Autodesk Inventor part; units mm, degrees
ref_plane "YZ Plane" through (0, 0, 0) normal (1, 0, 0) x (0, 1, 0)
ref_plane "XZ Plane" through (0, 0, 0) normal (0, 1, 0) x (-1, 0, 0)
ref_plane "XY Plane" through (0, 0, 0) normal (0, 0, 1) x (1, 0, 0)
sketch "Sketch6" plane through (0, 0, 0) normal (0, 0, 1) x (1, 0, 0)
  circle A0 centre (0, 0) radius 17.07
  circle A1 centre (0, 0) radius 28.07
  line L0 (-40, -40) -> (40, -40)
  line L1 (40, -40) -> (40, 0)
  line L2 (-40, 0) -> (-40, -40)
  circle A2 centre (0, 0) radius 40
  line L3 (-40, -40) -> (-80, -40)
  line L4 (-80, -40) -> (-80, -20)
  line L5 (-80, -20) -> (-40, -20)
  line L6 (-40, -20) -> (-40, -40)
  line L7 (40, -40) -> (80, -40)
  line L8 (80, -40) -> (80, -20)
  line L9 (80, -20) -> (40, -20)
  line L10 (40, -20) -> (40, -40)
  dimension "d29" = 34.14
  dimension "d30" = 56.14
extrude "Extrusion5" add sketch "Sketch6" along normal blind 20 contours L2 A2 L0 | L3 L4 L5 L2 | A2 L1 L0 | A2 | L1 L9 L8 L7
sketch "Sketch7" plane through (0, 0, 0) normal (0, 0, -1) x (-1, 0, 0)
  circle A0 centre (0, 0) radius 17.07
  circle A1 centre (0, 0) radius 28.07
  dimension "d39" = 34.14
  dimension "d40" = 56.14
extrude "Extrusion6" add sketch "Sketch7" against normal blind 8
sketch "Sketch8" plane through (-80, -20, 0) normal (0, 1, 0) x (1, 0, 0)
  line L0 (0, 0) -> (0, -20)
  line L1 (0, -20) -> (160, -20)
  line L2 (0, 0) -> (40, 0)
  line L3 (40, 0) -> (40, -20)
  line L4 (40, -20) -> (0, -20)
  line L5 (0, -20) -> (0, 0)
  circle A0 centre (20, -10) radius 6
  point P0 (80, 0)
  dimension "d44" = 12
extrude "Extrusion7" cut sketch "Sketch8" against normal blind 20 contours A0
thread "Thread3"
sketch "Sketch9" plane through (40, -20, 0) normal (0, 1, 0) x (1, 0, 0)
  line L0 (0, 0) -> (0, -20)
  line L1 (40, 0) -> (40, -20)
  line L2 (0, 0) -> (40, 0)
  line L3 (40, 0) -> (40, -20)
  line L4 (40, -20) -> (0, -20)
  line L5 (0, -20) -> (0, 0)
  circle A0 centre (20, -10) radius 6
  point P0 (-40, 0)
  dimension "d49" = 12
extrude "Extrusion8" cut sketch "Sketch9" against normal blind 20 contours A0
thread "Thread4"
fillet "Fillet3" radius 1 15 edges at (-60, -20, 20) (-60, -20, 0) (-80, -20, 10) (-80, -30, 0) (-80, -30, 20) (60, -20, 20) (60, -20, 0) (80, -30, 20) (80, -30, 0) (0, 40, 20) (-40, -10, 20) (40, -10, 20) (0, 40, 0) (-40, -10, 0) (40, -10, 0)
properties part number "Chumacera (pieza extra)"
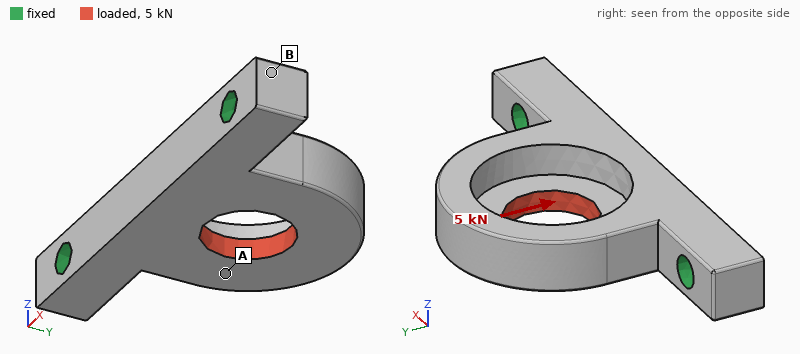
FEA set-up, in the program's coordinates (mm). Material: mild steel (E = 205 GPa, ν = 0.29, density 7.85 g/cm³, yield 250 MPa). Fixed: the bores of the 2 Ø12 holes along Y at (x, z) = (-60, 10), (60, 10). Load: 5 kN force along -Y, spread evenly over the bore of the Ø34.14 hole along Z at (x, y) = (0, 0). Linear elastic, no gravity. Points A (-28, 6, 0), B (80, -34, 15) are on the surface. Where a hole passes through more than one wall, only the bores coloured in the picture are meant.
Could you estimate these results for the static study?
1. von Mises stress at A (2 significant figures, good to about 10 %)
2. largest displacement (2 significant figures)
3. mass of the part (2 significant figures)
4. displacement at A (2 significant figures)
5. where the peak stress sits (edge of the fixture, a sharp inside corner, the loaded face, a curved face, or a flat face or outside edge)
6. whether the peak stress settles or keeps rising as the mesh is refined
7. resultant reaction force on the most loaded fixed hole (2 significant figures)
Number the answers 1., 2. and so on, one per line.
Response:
1. 10 MPa
2. 23 µm
3. 820 g
4. 12 µm
5. a sharp inside corner
6. keeps rising
7. 2.6 kN
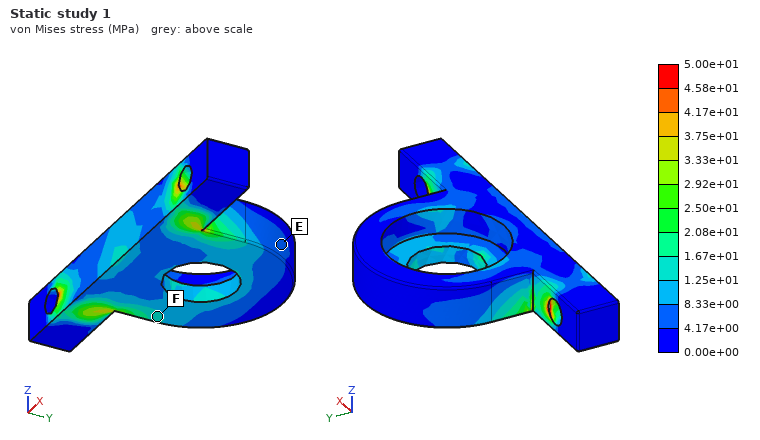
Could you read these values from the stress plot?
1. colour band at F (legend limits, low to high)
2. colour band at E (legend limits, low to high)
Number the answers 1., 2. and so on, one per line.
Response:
1. 1.25e+01 to 1.67e+01 MPa
2. 4.17e+00 to 8.33e+00 MPa
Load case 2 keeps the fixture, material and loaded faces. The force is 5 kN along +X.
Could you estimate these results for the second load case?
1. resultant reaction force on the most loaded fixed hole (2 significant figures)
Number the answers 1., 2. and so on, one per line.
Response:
1. 2.9 kN
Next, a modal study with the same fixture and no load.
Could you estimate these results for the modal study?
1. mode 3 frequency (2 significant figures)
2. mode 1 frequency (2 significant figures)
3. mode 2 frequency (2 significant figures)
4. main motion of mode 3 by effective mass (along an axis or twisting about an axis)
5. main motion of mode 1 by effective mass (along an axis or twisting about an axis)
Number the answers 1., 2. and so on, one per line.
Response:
1. 6400 Hz
2. 1900 Hz
3. 4900 Hz
4. along X
5. along Z
